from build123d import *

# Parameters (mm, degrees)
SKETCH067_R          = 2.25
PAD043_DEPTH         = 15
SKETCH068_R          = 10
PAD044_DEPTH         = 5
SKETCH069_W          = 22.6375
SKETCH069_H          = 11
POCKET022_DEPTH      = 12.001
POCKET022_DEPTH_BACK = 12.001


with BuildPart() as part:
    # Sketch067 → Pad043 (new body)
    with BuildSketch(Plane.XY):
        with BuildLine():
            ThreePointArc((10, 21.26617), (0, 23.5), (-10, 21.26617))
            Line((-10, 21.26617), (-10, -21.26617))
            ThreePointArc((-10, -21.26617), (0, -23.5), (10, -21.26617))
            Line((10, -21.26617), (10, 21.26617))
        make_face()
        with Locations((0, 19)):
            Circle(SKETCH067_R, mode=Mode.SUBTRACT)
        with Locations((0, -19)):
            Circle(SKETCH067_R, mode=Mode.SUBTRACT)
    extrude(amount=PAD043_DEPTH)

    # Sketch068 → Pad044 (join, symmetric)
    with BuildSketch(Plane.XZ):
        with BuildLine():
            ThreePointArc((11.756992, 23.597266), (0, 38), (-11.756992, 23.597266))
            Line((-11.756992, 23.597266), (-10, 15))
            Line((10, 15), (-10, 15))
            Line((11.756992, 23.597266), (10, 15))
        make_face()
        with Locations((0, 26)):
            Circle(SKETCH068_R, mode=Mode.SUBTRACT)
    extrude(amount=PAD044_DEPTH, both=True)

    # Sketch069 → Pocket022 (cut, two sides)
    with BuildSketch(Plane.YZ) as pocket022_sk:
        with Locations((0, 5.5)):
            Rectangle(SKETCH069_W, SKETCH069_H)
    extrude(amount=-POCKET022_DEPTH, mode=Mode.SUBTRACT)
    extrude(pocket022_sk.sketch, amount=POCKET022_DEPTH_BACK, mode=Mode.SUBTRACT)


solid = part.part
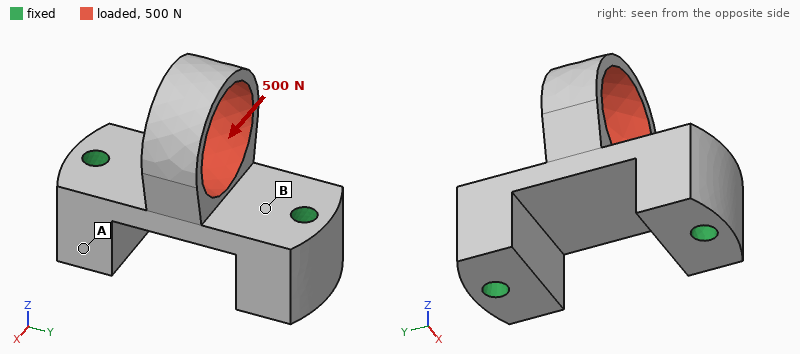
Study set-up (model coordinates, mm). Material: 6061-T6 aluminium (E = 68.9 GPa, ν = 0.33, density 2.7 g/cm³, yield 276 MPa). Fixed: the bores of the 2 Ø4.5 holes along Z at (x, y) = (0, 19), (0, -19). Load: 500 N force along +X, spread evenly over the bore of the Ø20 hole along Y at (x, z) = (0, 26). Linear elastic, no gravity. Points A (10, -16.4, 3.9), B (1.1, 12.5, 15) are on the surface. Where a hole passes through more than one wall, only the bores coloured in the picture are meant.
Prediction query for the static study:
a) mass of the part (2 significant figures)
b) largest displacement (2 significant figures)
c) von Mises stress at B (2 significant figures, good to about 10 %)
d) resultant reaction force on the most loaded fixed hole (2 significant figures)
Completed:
26 g
0.13 mm
19 MPa
250 N
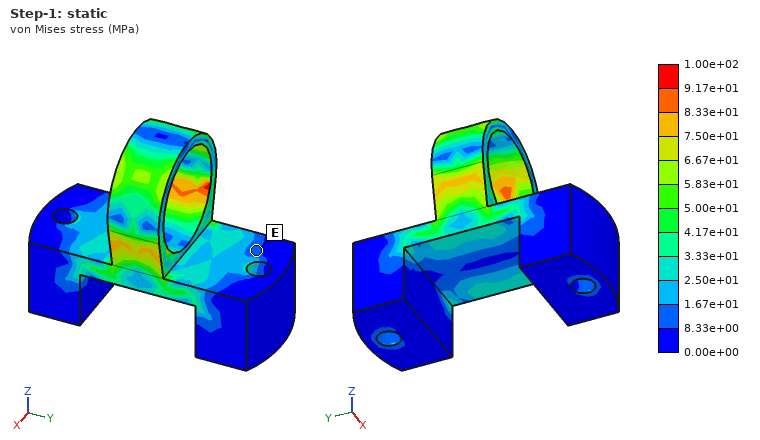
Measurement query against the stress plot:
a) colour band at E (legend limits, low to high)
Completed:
8.33e+00 to 1.67e+01 MPa
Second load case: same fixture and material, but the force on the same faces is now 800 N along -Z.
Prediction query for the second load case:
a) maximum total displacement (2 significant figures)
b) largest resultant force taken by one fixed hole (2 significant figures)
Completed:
37 µm
500 N
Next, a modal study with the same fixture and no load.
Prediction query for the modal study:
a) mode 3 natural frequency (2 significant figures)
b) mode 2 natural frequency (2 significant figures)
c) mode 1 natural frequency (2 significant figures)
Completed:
13 kHz
8100 Hz
5600 Hz
